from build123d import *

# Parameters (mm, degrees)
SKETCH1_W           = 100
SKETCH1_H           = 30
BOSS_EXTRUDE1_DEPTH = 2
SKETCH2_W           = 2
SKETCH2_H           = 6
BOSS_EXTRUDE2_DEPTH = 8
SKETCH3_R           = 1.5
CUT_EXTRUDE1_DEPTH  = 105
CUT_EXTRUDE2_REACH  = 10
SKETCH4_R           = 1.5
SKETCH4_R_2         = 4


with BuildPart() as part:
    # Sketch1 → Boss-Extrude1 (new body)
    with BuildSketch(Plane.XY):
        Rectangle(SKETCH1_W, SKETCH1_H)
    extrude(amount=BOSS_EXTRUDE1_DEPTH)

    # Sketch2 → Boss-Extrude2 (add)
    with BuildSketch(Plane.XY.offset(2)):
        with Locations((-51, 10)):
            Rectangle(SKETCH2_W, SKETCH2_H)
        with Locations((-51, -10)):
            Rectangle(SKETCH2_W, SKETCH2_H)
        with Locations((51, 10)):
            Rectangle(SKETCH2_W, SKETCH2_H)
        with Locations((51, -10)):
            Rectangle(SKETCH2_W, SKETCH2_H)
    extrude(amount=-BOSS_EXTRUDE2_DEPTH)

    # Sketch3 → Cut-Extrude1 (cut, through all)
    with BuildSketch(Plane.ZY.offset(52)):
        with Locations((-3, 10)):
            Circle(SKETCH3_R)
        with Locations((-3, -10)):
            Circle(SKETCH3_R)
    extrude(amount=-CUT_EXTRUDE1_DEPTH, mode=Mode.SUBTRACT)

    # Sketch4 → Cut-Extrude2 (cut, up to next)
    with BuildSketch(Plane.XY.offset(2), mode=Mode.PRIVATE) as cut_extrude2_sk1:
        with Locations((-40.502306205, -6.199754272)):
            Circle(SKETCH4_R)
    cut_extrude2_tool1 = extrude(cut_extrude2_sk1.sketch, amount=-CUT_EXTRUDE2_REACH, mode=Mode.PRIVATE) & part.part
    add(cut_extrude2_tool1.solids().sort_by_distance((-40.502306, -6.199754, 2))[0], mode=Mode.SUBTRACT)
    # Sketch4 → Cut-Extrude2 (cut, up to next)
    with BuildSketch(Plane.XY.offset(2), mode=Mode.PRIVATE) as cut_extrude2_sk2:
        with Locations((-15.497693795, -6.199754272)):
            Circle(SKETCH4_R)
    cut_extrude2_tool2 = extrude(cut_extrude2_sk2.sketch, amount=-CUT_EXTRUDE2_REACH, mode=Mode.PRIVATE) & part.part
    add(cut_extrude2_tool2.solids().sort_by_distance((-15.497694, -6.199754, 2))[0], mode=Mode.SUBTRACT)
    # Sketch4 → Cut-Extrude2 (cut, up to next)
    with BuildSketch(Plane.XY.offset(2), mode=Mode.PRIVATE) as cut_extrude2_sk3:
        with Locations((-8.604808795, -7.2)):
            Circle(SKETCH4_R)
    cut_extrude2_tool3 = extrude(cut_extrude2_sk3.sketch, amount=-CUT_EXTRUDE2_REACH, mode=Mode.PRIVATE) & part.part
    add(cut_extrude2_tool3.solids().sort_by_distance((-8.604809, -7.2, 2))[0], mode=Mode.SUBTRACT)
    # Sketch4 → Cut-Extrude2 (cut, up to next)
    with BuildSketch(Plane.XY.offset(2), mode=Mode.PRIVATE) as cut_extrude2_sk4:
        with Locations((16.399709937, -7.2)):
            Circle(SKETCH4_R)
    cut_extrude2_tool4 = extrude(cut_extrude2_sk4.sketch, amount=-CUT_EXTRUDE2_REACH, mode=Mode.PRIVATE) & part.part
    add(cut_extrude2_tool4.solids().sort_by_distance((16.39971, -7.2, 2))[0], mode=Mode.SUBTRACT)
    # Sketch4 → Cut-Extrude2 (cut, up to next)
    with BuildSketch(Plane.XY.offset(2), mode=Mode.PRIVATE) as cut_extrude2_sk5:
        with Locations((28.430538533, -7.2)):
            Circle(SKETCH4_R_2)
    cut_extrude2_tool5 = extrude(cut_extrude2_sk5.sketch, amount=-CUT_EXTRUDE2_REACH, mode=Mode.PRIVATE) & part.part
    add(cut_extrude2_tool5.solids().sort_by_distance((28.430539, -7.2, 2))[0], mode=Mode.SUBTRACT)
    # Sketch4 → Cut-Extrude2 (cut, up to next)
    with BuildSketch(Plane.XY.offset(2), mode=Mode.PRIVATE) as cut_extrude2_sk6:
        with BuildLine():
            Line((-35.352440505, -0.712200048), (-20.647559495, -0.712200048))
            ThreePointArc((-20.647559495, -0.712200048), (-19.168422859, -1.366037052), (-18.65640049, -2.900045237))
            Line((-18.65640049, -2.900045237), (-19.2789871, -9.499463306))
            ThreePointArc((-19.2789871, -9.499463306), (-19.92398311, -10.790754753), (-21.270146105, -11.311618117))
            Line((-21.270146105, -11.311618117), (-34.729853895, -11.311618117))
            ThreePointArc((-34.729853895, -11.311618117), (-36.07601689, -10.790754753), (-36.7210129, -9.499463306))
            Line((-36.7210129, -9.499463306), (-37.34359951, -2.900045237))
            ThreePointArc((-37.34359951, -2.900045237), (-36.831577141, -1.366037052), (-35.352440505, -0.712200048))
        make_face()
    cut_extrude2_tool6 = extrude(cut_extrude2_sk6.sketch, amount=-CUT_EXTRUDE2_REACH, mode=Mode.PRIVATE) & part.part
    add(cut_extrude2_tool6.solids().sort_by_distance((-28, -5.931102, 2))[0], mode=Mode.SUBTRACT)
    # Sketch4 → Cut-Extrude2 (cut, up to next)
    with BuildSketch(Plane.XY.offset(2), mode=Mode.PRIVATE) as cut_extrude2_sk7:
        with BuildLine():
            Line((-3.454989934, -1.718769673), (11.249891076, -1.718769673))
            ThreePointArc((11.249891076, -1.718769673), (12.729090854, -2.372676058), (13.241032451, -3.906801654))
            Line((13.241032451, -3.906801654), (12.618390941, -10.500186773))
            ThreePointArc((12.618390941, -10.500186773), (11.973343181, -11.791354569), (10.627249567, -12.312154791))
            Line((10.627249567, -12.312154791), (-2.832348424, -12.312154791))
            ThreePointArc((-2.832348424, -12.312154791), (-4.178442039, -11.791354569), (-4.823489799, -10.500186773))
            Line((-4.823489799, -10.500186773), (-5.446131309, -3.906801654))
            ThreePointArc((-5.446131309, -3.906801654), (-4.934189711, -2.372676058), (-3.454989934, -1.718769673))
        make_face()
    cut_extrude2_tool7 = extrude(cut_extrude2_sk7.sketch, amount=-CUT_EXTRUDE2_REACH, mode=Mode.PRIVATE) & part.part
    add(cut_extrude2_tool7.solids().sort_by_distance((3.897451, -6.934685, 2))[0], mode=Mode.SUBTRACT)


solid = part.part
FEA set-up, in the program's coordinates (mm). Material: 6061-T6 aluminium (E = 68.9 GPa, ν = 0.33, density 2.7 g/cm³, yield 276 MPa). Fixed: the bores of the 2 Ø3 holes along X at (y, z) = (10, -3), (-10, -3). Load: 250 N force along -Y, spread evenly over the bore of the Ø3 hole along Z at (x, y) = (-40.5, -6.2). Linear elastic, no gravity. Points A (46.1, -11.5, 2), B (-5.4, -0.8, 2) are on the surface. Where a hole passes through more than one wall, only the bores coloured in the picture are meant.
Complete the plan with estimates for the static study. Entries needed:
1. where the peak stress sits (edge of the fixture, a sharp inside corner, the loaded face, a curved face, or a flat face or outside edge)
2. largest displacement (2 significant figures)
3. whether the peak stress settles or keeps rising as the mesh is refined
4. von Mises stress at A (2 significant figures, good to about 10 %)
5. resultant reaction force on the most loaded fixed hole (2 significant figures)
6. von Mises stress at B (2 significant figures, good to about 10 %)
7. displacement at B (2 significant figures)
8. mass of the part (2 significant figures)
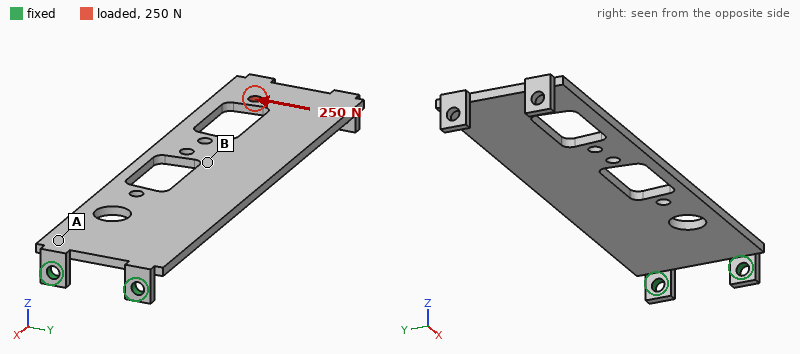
edge of the fixture
0.80 mm
keeps rising
58 MPa
1.1 kN
28 MPa
0.33 mm
15 g
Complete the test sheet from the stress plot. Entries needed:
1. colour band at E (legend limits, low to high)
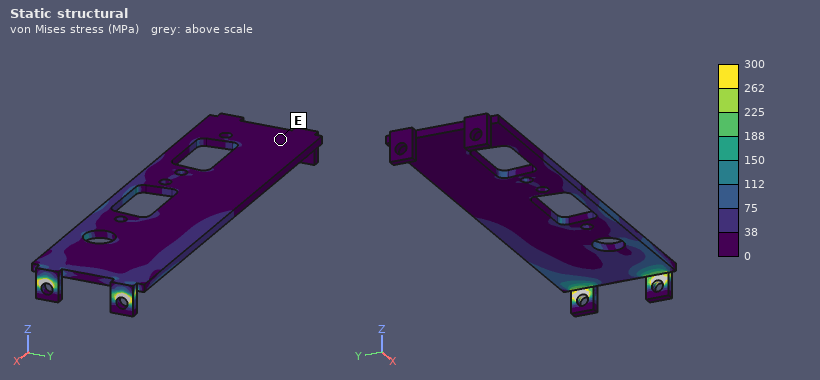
0 to 38 MPa
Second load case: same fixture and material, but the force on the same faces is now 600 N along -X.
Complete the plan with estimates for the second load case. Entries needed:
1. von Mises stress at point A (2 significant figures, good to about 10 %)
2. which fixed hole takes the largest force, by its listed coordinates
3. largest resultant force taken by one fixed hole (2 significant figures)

25 MPa
(-10, -3)
480 N
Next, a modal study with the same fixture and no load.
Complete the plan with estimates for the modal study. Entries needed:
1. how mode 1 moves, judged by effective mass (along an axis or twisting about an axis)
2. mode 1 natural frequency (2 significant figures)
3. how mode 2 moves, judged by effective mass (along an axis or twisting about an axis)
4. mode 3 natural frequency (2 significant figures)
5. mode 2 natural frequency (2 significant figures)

along Z
130 Hz
along Z
950 Hz
800 Hz
